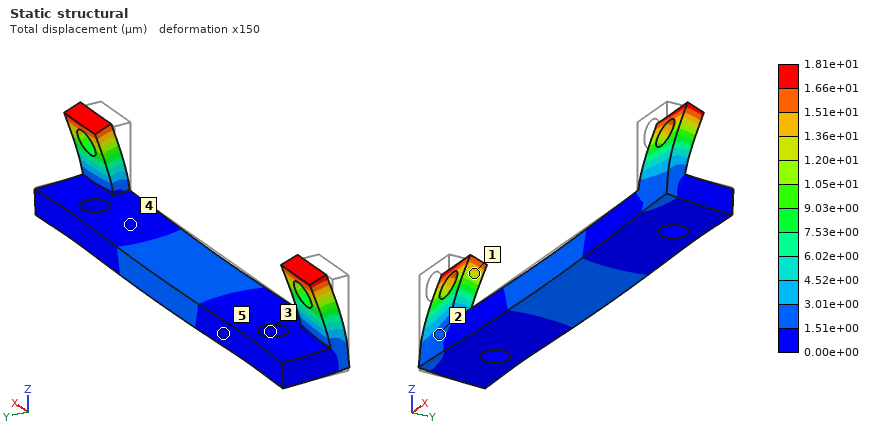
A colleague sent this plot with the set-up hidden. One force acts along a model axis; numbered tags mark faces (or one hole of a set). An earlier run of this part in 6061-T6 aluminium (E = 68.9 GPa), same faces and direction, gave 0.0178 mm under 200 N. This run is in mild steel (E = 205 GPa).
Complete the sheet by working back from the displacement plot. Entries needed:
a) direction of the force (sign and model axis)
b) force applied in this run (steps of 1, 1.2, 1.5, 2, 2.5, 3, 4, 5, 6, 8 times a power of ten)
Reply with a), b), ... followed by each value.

a) +Y
b) 600 N
